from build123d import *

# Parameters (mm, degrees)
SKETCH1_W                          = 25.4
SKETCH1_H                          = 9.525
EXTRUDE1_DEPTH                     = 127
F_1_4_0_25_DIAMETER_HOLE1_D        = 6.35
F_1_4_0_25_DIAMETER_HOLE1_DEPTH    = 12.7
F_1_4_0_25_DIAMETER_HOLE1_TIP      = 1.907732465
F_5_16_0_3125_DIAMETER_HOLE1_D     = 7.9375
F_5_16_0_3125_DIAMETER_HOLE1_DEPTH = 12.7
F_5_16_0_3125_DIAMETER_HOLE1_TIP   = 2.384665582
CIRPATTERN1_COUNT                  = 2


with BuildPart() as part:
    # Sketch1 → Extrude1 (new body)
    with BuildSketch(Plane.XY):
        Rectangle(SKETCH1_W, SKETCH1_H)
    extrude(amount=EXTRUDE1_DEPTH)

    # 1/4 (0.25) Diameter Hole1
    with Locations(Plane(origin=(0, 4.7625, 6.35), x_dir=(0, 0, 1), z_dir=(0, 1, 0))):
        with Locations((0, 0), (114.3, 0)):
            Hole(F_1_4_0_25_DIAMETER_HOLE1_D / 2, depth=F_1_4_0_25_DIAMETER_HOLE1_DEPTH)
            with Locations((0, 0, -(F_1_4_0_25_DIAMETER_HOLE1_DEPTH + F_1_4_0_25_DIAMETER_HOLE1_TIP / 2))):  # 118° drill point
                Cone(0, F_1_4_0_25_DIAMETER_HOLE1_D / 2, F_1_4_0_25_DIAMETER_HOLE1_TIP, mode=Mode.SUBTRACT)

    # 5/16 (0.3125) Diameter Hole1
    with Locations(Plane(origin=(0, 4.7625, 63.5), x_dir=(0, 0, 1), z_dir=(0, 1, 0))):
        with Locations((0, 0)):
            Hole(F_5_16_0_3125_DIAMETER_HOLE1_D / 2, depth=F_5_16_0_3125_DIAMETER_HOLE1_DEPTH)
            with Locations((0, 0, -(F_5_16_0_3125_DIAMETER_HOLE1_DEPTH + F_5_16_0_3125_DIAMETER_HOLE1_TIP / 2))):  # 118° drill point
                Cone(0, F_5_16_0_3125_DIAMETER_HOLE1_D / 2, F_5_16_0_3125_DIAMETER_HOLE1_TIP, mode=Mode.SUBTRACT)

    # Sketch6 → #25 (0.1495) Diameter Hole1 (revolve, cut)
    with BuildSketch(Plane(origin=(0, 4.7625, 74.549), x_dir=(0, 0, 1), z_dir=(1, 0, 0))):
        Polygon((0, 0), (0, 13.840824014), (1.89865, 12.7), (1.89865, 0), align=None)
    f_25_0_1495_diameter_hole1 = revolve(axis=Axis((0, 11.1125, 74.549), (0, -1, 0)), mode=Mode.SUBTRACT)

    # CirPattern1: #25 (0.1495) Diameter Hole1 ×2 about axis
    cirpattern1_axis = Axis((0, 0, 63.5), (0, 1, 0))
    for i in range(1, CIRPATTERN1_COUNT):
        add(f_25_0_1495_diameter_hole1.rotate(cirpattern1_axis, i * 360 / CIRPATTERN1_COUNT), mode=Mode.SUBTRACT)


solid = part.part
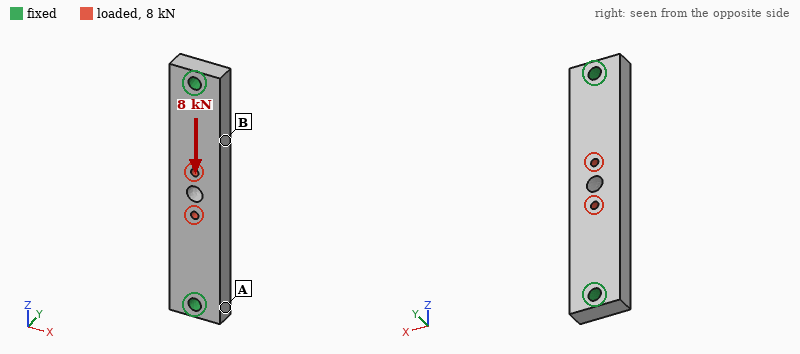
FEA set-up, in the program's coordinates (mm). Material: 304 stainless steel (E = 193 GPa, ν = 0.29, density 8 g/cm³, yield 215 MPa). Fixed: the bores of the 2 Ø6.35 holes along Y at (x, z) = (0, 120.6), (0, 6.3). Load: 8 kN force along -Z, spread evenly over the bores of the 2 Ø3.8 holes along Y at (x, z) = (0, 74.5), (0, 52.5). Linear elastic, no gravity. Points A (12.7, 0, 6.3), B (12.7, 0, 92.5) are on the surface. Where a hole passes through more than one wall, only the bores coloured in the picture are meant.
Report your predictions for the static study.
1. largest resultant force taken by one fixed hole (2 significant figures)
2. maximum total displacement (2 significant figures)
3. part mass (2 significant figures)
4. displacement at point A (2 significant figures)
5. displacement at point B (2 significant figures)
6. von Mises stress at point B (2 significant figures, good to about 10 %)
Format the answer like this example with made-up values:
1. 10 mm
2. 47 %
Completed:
1. 4.0 kN
2. 5.5 µm
3. 240 g
4. 1.2 µm
5. 2.9 µm
6. 16 MPa
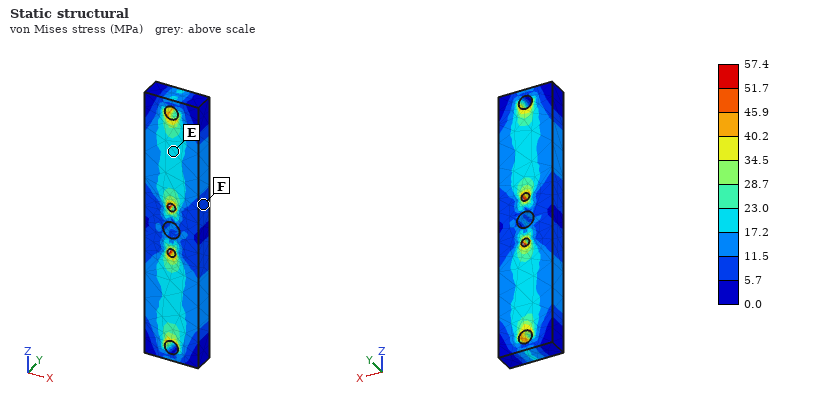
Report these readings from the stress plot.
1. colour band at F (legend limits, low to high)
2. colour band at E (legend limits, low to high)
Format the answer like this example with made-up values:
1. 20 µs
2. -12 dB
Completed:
1. 5.7 to 11.5 MPa
2. 17.2 to 23.0 MPa
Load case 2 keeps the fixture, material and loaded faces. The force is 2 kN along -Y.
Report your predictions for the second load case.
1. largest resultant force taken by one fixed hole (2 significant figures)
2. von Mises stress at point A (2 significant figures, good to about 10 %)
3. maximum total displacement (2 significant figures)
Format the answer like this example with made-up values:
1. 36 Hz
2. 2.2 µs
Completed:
1. 1.0 kN
2. 15 MPa
3. 47 µm
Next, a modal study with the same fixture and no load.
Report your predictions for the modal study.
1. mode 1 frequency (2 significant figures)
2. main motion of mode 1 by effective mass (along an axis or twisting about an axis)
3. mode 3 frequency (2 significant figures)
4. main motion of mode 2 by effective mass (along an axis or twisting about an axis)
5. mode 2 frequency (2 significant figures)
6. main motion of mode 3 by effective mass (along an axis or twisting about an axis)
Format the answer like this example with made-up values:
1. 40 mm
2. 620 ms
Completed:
1. 3500 Hz
2. along Y
3. 8300 Hz
4. along X
5. 6000 Hz
6. twisting about Z
